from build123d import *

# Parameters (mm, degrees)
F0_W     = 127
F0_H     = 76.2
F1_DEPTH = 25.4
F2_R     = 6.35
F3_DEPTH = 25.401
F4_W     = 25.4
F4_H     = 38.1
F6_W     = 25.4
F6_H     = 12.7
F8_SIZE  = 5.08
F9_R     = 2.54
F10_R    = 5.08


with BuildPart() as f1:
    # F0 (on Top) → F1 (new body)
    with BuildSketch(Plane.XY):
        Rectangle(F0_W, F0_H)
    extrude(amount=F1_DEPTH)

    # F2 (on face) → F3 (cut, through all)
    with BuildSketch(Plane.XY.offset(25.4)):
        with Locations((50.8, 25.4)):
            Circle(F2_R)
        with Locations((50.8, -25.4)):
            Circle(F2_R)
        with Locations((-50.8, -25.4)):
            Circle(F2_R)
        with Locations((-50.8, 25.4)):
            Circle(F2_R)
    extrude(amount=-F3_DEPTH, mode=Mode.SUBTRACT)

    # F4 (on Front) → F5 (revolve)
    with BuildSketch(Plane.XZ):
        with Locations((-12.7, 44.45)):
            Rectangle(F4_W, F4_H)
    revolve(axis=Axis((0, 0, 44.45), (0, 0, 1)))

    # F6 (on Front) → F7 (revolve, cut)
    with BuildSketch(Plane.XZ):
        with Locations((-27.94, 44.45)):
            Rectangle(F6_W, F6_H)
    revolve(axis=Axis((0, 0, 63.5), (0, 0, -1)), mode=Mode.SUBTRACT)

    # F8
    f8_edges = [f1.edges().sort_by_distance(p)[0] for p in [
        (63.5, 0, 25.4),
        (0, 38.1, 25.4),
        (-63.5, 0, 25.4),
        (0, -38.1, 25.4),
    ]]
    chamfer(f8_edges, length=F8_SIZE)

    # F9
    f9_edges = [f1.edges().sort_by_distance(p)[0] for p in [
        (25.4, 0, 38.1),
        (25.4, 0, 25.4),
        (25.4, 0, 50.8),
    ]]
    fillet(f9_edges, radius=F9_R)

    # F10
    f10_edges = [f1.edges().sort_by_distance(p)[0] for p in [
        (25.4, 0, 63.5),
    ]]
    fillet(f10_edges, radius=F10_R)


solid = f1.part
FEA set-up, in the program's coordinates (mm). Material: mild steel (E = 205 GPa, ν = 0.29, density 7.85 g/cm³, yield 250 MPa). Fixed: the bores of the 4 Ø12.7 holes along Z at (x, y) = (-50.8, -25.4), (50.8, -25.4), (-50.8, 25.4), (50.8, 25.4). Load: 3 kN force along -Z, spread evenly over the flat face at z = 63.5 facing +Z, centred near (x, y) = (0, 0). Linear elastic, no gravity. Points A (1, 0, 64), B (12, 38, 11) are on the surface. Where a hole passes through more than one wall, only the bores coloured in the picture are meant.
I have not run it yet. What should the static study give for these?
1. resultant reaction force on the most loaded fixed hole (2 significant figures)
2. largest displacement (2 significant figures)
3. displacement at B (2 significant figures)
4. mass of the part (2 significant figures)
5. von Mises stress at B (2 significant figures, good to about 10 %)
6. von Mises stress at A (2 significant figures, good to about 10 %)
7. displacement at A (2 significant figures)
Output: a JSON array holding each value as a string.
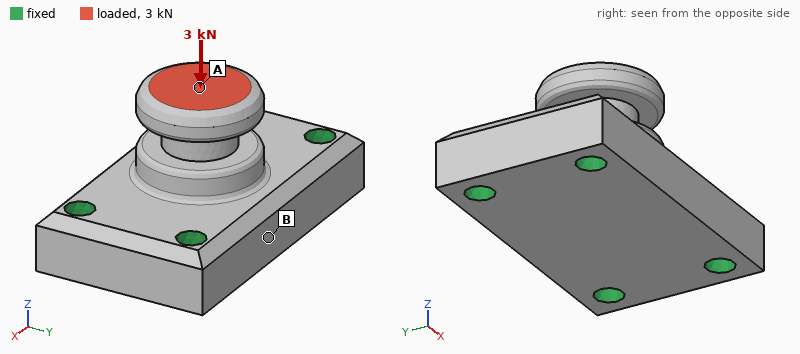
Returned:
["780 N", "1.5 µm", "0.71 µm", "2.3 kg", "0.95 MPa", "3.9 MPa", "1.4 µm"]
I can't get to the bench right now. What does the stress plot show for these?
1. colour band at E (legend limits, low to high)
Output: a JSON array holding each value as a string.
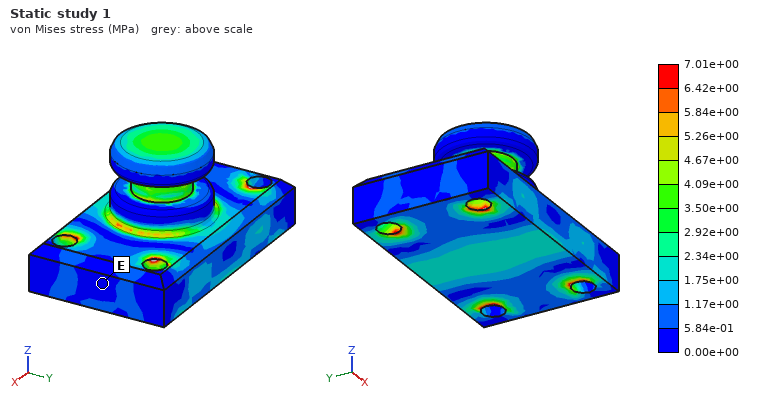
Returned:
["0.00e+00 to 5.84e-01 MPa"]
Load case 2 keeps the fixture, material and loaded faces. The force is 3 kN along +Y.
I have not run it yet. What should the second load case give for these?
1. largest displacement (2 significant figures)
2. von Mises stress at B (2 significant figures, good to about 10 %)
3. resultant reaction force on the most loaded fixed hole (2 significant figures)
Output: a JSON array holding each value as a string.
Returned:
["10 µm", "3.8 MPa", "1.7 kN"]
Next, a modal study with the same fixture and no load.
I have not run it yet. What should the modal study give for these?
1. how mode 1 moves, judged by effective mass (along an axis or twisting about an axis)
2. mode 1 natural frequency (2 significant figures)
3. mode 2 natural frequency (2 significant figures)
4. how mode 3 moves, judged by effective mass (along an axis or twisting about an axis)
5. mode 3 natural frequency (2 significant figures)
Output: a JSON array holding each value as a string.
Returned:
["along Y", "6500 Hz", "8100 Hz", "along Z", "8400 Hz"]
